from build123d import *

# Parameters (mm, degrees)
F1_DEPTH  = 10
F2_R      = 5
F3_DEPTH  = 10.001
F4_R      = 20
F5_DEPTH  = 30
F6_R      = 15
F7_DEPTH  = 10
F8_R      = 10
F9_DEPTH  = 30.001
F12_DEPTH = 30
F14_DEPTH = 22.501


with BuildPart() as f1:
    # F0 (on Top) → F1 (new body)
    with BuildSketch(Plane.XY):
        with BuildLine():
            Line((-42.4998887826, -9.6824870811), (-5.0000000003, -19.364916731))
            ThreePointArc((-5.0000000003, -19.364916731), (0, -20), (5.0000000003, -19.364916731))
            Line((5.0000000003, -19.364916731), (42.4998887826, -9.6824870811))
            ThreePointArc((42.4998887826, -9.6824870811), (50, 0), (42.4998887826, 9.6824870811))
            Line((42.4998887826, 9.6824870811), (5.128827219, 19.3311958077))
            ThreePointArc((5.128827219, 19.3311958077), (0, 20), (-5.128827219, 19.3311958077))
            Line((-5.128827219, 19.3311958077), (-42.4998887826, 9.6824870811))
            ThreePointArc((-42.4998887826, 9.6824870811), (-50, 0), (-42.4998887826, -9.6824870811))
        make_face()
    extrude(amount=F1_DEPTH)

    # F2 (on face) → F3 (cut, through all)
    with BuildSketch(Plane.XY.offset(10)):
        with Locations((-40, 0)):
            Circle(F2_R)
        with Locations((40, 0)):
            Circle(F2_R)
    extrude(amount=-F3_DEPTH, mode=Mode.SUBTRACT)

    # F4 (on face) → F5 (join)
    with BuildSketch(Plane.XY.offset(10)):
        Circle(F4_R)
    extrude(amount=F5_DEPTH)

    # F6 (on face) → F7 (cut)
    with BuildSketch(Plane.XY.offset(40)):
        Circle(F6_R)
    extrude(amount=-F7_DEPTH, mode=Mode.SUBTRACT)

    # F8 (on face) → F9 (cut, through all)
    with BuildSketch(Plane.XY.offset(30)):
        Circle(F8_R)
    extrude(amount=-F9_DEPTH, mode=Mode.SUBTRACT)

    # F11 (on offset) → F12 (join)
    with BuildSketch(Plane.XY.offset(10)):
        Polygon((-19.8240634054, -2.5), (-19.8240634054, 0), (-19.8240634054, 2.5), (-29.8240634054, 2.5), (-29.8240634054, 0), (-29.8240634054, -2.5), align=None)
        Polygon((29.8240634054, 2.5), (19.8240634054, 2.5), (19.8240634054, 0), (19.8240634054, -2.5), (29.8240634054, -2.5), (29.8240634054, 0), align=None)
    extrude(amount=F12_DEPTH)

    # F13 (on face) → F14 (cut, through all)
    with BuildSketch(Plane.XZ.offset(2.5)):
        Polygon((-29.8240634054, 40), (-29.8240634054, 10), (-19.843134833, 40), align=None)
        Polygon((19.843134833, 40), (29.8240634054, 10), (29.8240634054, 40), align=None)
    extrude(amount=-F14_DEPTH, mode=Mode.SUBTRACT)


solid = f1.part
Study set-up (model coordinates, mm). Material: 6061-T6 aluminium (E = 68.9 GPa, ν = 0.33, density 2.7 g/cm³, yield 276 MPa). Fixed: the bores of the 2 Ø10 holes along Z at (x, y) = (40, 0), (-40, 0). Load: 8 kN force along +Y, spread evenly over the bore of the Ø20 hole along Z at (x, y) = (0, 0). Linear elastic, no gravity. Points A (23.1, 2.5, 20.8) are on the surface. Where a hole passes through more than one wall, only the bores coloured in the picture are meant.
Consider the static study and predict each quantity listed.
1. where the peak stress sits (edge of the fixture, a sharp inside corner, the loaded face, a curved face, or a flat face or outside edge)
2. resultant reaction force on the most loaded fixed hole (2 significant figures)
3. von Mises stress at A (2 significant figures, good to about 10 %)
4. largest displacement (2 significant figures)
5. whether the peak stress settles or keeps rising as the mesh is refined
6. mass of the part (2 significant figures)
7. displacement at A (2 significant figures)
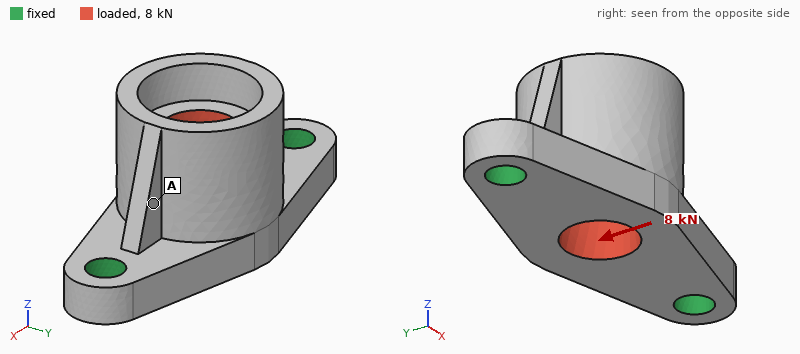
edge of the fixture
4.0 kN
28 MPa
0.18 mm
keeps rising
130 g
0.082 mm
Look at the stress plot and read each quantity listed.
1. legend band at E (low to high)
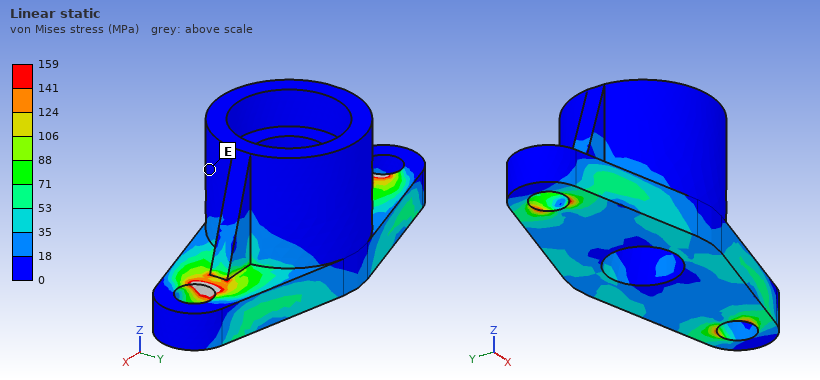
0 to 18 MPa
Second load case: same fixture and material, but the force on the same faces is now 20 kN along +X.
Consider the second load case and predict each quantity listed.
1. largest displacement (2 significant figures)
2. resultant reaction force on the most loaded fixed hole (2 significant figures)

38 µm
10 kN
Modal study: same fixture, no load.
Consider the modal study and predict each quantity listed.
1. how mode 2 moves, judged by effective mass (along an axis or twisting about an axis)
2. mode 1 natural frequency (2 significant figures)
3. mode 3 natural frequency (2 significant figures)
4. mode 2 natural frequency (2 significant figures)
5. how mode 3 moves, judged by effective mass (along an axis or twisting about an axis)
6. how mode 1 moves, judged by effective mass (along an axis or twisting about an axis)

along Z
3400 Hz
11 kHz
7200 Hz
along X
along Y
